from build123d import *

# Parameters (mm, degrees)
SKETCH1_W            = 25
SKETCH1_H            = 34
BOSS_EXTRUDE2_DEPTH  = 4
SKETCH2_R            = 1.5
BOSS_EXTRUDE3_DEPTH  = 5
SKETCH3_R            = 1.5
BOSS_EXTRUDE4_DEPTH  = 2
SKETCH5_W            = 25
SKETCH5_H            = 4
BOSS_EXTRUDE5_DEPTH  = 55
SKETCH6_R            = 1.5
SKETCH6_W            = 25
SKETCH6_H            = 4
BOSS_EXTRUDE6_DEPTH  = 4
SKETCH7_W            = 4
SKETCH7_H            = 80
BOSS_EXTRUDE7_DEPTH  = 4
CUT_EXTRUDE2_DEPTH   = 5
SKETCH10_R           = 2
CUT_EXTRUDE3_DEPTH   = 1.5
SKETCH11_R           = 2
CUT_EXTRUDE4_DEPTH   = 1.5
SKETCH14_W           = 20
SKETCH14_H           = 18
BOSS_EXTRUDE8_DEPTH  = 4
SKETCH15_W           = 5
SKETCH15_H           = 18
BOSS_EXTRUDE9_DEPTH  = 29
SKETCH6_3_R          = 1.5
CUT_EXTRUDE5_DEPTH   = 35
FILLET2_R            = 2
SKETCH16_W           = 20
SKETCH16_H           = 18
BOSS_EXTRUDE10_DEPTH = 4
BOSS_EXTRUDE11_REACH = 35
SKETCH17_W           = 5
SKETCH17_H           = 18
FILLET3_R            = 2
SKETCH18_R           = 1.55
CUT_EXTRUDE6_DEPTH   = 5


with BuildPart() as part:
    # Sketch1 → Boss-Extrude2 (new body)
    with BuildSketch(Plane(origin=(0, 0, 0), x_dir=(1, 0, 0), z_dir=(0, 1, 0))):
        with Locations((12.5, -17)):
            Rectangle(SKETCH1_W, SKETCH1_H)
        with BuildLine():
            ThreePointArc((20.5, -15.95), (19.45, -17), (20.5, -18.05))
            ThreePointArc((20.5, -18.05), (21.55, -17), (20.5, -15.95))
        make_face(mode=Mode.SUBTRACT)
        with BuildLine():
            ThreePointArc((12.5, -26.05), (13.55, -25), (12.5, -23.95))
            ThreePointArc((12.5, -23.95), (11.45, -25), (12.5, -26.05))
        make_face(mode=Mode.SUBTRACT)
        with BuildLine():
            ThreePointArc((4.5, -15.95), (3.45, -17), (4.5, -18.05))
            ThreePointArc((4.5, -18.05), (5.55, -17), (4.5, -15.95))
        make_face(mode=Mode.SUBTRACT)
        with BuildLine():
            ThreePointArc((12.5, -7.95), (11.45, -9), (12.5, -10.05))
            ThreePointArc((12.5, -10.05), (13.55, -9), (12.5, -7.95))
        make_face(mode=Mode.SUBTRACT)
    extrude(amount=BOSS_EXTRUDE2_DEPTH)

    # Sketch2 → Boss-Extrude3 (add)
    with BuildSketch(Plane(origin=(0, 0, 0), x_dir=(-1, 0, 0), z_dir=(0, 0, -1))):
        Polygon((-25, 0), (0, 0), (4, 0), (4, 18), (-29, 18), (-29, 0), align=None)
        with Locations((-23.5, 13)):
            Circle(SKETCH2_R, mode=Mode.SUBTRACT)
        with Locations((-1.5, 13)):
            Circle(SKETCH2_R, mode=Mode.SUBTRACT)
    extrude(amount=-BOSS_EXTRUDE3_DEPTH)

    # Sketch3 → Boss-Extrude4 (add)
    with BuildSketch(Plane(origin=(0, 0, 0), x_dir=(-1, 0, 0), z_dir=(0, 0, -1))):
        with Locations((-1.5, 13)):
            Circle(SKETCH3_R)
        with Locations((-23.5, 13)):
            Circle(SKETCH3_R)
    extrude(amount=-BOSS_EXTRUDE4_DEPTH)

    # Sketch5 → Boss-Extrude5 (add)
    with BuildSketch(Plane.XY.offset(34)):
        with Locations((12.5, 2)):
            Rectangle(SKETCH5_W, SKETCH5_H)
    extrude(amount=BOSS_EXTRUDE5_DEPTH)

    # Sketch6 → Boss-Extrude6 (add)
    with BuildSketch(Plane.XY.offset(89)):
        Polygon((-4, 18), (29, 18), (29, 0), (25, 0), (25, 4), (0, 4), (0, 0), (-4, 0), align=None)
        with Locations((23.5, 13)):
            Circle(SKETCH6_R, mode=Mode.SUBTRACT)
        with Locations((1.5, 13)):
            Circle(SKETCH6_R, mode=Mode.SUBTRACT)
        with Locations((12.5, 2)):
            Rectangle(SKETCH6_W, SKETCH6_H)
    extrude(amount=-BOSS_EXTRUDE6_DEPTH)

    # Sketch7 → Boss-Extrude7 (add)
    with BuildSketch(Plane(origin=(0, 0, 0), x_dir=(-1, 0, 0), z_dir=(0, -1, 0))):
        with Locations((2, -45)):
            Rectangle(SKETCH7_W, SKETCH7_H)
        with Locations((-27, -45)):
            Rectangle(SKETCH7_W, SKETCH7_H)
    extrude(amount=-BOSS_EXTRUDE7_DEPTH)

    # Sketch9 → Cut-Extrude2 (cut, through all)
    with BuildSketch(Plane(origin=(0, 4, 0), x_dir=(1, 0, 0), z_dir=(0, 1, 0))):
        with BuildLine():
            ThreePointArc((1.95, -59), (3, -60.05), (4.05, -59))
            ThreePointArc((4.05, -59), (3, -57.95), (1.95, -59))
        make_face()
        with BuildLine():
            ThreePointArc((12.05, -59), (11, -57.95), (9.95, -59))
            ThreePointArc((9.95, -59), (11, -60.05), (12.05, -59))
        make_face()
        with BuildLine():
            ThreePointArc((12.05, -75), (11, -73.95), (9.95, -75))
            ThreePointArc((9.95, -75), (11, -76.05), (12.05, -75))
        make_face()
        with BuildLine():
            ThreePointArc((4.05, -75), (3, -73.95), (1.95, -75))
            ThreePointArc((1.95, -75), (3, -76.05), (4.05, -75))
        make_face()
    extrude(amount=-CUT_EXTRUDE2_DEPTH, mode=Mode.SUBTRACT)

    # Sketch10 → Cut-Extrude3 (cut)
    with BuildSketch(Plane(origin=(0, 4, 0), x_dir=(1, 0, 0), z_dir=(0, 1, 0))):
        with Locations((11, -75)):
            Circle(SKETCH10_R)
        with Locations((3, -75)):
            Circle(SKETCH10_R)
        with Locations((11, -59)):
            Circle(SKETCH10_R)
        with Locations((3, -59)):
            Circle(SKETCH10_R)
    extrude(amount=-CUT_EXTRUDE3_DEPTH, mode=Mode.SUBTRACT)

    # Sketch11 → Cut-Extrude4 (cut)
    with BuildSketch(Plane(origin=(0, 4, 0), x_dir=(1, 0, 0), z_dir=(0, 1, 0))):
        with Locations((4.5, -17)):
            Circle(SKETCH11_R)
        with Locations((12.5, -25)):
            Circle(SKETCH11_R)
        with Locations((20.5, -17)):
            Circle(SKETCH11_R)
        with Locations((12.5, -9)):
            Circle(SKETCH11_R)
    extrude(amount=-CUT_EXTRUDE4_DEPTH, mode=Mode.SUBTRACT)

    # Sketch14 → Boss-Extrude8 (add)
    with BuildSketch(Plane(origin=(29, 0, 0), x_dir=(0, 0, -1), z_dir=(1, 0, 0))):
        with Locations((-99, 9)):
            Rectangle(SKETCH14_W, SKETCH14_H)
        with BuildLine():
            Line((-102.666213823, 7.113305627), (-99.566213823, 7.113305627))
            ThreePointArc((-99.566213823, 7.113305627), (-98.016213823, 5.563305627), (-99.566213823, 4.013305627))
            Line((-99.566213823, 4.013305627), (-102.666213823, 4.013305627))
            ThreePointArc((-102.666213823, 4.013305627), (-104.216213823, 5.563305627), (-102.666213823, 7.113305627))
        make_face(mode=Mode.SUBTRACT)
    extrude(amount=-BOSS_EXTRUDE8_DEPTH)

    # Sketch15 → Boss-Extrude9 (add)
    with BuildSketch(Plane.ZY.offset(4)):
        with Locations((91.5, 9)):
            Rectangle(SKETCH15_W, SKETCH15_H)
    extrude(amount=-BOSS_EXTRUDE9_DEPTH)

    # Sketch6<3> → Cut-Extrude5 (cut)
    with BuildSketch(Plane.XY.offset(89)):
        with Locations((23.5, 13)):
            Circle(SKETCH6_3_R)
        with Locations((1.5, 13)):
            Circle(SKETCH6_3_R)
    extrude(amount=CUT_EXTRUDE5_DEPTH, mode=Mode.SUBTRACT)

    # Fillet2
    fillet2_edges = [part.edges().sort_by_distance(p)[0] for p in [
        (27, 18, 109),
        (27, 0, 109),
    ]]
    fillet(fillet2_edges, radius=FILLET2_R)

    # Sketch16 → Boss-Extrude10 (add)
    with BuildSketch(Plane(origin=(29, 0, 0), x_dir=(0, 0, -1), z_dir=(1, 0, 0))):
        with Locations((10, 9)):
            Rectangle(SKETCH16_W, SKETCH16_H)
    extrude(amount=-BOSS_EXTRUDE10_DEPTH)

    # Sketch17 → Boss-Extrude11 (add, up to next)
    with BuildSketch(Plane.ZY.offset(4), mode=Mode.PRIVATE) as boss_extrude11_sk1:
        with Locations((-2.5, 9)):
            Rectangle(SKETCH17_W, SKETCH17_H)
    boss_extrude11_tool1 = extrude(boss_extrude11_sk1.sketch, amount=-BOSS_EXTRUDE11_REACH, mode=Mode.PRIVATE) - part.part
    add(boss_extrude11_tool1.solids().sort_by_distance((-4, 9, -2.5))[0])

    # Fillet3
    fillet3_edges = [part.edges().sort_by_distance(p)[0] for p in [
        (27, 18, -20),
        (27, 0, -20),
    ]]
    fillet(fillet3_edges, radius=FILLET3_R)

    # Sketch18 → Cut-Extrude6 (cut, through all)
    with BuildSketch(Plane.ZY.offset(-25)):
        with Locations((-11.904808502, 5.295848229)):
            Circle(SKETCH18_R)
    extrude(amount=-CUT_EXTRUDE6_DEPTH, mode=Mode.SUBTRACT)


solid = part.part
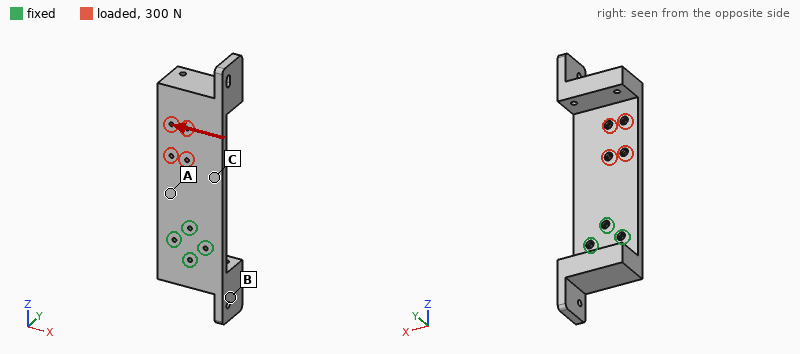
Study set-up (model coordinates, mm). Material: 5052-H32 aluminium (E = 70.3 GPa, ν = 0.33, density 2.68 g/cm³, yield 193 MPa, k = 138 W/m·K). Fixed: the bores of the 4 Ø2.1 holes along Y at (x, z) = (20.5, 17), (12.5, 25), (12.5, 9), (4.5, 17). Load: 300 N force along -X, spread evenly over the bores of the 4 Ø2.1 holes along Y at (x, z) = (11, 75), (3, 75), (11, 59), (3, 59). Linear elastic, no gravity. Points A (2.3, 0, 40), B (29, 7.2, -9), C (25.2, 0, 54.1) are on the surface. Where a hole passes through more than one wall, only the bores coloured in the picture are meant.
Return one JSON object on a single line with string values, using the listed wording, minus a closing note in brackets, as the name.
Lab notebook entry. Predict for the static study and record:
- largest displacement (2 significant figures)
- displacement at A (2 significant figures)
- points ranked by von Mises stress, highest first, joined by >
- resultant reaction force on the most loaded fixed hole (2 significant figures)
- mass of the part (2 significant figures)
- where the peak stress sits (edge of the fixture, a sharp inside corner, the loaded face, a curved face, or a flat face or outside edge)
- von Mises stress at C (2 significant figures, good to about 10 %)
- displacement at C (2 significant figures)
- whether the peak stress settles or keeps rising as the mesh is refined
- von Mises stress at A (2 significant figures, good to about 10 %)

{"largest displacement": "52 µm", "displacement at A": "9.8 µm", "points ranked by von Mises stress, highest first, joined by >": "A > C > B", "resultant reaction force on the most loaded fixed hole": "530 N", "mass of the part": "63 g", "where the peak stress sits": "edge of the fixture", "von Mises stress at C": "6.0 MPa", "displacement at C": "19 µm", "whether the peak stress settles or keeps rising as the mesh is refined": "keeps rising", "von Mises stress at A": "9.0 MPa"}
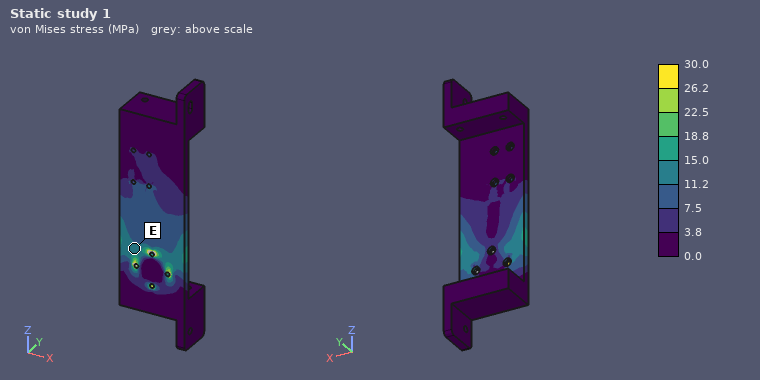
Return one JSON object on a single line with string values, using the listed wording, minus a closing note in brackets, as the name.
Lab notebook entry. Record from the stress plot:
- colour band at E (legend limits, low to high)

{"colour band at E": "11.2 to 15.0 MPa"}
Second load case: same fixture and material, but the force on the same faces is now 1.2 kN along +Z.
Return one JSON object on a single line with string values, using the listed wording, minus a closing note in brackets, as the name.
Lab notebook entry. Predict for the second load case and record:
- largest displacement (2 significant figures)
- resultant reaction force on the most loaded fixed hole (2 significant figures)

{"largest displacement": "0.20 mm", "resultant reaction force on the most loaded fixed hole": "540 N"}
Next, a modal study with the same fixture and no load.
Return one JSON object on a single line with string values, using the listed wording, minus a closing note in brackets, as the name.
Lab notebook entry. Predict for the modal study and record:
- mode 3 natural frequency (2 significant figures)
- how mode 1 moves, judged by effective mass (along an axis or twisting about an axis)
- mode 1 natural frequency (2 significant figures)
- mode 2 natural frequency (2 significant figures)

{"mode 3 natural frequency": "2300 Hz", "how mode 1 moves, judged by effective mass": "along Y", "mode 1 natural frequency": "360 Hz", "mode 2 natural frequency": "1300 Hz"}
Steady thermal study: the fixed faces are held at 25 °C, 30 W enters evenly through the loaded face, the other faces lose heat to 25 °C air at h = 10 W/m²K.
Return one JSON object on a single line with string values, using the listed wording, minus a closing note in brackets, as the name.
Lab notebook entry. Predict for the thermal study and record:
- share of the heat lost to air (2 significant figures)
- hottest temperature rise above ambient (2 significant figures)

{"share of the heat lost to air": "14 %", "hottest temperature rise above ambient": "76 K"}
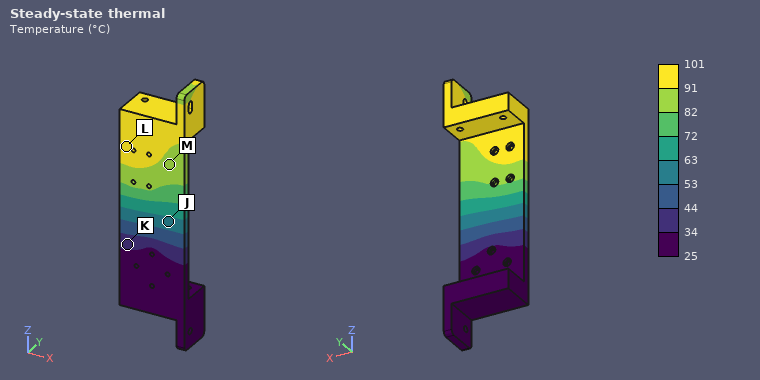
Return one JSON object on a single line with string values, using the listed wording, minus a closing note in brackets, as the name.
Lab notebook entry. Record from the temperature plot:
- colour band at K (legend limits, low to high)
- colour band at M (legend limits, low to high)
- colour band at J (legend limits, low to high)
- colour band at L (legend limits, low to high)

{"colour band at K": "34 to 44 °C", "colour band at M": "82 to 91 °C", "colour band at J": "53 to 63 °C", "colour band at L": "91 to 101 °C"}
